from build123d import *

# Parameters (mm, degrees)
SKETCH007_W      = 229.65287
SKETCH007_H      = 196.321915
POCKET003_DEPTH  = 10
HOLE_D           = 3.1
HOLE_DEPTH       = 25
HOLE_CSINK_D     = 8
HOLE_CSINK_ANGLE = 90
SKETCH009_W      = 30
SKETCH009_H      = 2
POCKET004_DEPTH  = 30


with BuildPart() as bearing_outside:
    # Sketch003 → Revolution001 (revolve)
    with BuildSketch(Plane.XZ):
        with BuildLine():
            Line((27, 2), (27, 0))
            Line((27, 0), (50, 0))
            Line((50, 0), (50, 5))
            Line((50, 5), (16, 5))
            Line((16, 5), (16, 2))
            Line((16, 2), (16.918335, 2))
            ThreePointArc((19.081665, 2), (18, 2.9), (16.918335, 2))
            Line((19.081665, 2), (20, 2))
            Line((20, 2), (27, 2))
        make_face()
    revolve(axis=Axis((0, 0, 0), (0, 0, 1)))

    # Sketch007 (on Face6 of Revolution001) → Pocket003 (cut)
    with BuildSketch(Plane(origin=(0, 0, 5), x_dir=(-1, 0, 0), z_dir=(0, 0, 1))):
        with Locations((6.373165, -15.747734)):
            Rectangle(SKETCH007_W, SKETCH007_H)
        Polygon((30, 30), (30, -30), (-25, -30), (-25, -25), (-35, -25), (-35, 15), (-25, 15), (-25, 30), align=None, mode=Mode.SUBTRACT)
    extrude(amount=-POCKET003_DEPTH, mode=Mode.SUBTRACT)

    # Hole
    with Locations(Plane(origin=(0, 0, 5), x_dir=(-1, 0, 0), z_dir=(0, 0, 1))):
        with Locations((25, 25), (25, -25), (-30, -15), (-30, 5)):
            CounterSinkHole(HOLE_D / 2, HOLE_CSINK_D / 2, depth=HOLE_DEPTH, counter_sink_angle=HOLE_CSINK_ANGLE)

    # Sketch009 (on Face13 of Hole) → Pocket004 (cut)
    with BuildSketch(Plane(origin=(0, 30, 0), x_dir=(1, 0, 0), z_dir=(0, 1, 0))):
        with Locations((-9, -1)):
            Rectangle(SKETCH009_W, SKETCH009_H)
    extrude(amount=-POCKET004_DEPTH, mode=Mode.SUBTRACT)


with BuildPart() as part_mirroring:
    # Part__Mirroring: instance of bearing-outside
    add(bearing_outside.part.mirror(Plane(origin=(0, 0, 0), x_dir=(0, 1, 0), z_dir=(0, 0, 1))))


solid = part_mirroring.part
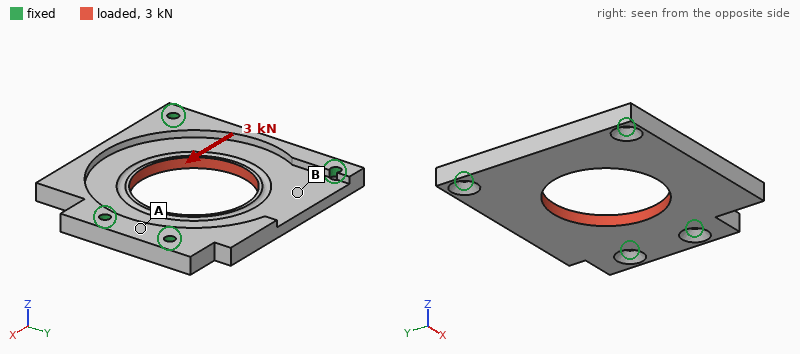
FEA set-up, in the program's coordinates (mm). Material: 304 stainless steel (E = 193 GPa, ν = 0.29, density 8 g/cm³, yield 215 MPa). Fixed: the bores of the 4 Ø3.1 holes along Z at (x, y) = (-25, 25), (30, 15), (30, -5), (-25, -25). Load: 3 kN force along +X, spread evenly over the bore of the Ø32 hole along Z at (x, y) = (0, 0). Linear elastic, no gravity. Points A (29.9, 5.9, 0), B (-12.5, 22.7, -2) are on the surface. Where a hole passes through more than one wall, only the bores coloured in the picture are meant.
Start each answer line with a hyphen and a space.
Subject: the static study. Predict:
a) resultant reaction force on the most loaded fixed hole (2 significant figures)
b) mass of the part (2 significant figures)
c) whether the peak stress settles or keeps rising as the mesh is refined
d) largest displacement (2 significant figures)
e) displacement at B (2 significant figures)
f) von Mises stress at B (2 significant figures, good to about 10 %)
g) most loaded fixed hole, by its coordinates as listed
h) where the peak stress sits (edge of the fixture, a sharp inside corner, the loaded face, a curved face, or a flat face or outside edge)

- 1.0 kN
- 85 g
- keeps rising
- 9.2 µm
- 3.8 µm
- 17 MPa
- (-25, -25)
- edge of the fixture
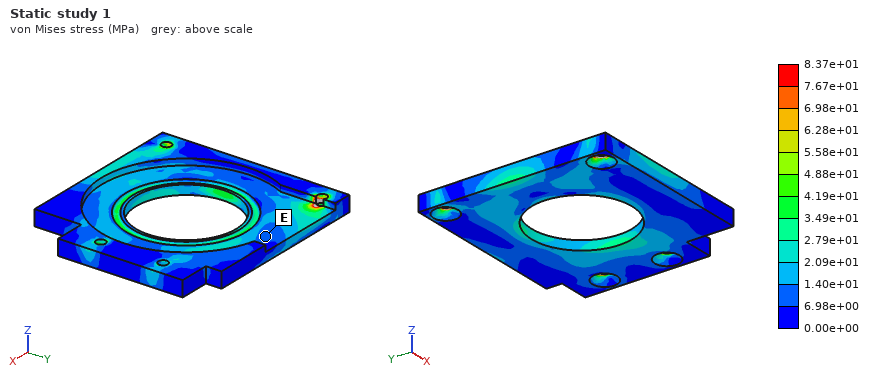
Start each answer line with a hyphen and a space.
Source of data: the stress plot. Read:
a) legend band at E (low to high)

- 6.98e+00 to 1.40e+01 MPa
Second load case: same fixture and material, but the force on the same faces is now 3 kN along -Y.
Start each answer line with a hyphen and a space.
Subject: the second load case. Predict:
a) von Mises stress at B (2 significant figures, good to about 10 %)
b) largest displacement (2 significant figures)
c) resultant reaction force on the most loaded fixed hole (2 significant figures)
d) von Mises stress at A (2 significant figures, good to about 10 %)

- 13 MPa
- 7.7 µm
- 830 N
- 12 MPa
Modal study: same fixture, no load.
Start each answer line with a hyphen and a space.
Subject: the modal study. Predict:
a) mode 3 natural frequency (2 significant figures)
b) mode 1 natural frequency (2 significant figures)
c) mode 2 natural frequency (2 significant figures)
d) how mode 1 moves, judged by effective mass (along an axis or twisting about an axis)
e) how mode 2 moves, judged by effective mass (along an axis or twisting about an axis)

- 7000 Hz
- 4400 Hz
- 5000 Hz
- along Z
- along Z
